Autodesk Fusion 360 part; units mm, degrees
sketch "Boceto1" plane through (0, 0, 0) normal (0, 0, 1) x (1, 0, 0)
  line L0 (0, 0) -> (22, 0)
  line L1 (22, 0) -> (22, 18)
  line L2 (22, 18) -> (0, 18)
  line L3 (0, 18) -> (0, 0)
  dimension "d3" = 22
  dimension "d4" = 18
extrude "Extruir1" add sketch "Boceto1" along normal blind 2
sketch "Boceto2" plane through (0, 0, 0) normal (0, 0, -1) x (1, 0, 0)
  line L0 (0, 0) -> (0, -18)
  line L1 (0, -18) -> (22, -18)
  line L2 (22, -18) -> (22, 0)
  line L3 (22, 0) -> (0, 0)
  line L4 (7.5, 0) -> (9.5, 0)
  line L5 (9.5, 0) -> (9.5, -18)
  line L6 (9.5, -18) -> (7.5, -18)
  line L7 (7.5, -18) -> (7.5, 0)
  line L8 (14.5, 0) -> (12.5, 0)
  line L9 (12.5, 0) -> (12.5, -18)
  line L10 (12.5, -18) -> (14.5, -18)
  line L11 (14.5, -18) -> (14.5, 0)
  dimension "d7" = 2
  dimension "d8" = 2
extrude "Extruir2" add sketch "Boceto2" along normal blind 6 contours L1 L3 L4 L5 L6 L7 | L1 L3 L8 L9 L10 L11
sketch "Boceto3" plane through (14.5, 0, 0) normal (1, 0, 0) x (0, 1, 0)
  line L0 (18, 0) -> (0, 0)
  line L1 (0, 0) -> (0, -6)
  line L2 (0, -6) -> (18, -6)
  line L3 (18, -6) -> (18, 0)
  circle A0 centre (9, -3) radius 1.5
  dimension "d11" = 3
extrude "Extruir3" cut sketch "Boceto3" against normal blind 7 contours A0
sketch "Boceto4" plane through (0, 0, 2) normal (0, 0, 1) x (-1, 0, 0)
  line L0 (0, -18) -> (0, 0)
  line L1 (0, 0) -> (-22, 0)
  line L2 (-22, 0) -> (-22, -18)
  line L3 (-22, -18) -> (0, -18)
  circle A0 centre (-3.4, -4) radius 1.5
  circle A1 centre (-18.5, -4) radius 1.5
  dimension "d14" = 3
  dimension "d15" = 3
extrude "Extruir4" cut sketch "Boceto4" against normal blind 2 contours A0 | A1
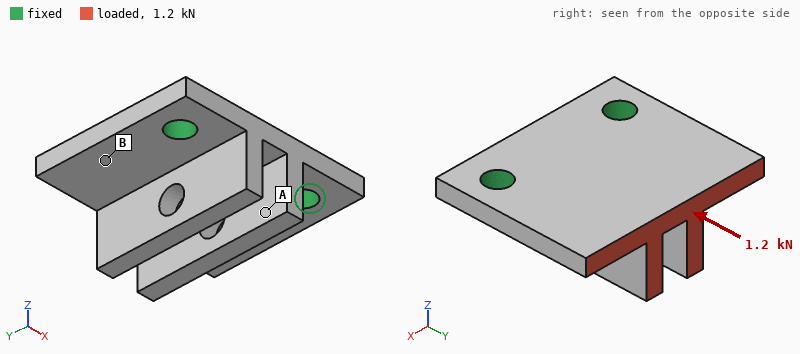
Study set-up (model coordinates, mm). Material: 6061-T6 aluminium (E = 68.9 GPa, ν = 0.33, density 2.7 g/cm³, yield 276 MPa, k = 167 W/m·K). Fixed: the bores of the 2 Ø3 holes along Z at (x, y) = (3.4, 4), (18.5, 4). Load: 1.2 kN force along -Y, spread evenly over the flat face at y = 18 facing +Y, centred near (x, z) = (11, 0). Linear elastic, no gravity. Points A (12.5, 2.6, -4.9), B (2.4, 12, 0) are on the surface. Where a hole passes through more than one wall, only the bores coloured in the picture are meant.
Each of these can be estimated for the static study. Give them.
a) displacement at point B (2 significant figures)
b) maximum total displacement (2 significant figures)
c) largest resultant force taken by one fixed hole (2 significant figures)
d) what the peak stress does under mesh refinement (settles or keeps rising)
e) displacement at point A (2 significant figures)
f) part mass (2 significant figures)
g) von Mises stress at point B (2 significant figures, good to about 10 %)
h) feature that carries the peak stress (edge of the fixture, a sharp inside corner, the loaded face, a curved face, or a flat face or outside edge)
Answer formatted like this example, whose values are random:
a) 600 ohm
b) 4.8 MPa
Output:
a) 20 µm
b) 59 µm
c) 610 N
d) keeps rising
e) 24 µm
f) 3.2 g
g) 33 MPa
h) edge of the fixture
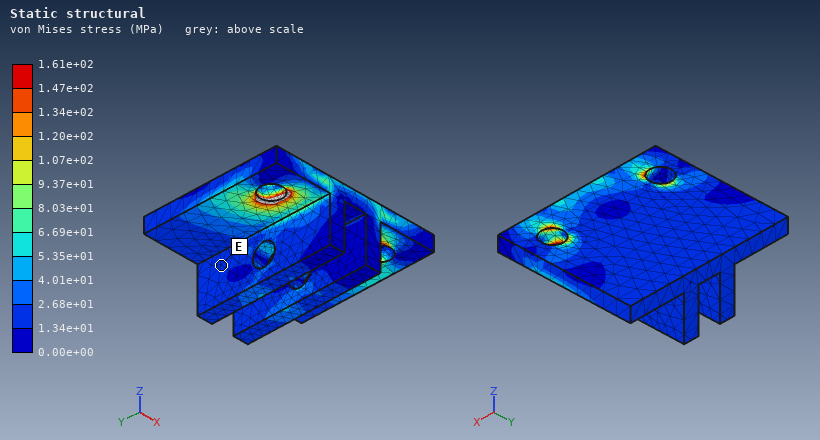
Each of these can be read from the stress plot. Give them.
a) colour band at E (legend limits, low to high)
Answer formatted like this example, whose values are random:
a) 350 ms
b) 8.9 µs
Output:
a) 1.34e+01 to 2.68e+01 MPa
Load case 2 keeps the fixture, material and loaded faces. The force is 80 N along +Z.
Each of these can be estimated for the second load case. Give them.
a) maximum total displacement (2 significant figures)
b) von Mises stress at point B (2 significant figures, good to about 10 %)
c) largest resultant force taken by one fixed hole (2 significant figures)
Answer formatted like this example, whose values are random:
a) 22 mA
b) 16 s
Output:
a) 36 µm
b) 9.5 MPa
c) 42 N
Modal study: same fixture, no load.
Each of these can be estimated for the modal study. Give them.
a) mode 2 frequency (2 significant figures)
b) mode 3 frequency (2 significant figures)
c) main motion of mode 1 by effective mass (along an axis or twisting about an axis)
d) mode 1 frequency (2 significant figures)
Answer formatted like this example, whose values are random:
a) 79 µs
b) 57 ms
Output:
a) 16 kHz
b) 22 kHz
c) along Z
d) 8500 Hz
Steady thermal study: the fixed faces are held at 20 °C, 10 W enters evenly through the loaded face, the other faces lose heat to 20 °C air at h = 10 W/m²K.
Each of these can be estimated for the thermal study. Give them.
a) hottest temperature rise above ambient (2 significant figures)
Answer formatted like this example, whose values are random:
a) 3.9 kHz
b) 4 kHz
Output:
a) 16 K
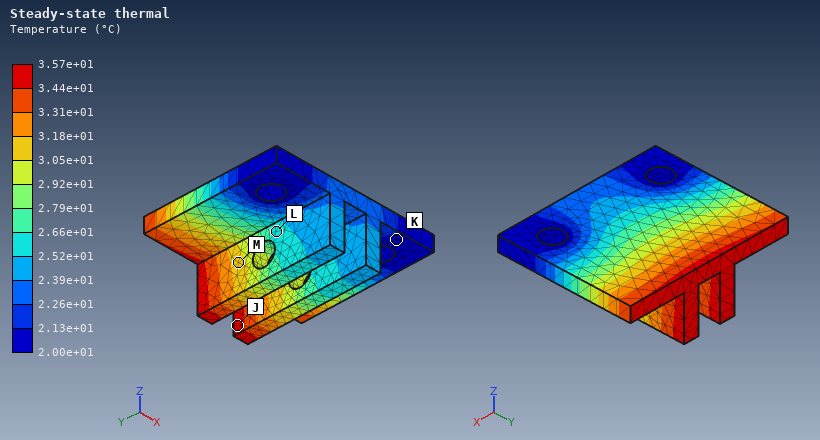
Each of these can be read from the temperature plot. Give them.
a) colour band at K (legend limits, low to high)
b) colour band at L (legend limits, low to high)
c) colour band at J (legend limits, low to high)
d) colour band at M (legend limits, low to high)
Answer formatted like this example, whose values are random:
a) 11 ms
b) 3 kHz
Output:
a) 2.00e+01 to 2.13e+01 °C
b) 2.52e+01 to 2.66e+01 °C
c) 3.44e+01 to 3.57e+01 °C
d) 3.05e+01 to 3.18e+01 °C
